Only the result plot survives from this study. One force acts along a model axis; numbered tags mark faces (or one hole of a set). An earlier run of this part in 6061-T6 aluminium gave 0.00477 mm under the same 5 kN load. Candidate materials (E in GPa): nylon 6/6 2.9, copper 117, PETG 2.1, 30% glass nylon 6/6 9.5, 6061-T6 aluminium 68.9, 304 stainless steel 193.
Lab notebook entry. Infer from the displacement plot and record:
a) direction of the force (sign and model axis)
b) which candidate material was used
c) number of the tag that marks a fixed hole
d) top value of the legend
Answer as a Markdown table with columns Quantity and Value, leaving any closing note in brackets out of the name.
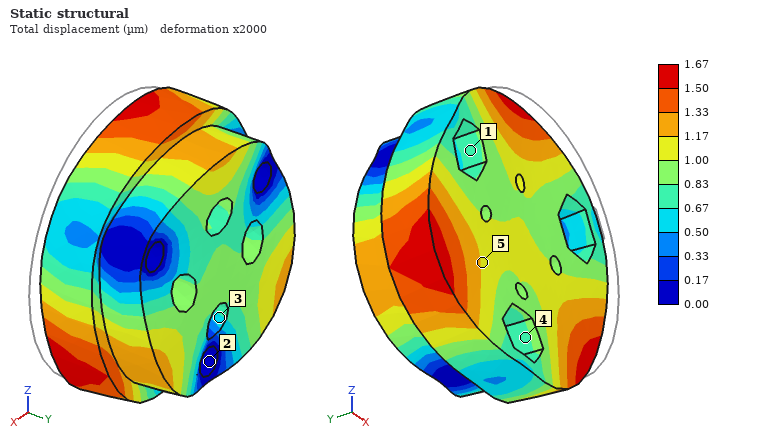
| Quantity | Value |
|---|---|
| direction of the force | +Y |
| which candidate material was used | 304 stainless steel |
| number of the tag that marks a fixed hole | 2 |
| top value of the legend | 1.67 µm |
